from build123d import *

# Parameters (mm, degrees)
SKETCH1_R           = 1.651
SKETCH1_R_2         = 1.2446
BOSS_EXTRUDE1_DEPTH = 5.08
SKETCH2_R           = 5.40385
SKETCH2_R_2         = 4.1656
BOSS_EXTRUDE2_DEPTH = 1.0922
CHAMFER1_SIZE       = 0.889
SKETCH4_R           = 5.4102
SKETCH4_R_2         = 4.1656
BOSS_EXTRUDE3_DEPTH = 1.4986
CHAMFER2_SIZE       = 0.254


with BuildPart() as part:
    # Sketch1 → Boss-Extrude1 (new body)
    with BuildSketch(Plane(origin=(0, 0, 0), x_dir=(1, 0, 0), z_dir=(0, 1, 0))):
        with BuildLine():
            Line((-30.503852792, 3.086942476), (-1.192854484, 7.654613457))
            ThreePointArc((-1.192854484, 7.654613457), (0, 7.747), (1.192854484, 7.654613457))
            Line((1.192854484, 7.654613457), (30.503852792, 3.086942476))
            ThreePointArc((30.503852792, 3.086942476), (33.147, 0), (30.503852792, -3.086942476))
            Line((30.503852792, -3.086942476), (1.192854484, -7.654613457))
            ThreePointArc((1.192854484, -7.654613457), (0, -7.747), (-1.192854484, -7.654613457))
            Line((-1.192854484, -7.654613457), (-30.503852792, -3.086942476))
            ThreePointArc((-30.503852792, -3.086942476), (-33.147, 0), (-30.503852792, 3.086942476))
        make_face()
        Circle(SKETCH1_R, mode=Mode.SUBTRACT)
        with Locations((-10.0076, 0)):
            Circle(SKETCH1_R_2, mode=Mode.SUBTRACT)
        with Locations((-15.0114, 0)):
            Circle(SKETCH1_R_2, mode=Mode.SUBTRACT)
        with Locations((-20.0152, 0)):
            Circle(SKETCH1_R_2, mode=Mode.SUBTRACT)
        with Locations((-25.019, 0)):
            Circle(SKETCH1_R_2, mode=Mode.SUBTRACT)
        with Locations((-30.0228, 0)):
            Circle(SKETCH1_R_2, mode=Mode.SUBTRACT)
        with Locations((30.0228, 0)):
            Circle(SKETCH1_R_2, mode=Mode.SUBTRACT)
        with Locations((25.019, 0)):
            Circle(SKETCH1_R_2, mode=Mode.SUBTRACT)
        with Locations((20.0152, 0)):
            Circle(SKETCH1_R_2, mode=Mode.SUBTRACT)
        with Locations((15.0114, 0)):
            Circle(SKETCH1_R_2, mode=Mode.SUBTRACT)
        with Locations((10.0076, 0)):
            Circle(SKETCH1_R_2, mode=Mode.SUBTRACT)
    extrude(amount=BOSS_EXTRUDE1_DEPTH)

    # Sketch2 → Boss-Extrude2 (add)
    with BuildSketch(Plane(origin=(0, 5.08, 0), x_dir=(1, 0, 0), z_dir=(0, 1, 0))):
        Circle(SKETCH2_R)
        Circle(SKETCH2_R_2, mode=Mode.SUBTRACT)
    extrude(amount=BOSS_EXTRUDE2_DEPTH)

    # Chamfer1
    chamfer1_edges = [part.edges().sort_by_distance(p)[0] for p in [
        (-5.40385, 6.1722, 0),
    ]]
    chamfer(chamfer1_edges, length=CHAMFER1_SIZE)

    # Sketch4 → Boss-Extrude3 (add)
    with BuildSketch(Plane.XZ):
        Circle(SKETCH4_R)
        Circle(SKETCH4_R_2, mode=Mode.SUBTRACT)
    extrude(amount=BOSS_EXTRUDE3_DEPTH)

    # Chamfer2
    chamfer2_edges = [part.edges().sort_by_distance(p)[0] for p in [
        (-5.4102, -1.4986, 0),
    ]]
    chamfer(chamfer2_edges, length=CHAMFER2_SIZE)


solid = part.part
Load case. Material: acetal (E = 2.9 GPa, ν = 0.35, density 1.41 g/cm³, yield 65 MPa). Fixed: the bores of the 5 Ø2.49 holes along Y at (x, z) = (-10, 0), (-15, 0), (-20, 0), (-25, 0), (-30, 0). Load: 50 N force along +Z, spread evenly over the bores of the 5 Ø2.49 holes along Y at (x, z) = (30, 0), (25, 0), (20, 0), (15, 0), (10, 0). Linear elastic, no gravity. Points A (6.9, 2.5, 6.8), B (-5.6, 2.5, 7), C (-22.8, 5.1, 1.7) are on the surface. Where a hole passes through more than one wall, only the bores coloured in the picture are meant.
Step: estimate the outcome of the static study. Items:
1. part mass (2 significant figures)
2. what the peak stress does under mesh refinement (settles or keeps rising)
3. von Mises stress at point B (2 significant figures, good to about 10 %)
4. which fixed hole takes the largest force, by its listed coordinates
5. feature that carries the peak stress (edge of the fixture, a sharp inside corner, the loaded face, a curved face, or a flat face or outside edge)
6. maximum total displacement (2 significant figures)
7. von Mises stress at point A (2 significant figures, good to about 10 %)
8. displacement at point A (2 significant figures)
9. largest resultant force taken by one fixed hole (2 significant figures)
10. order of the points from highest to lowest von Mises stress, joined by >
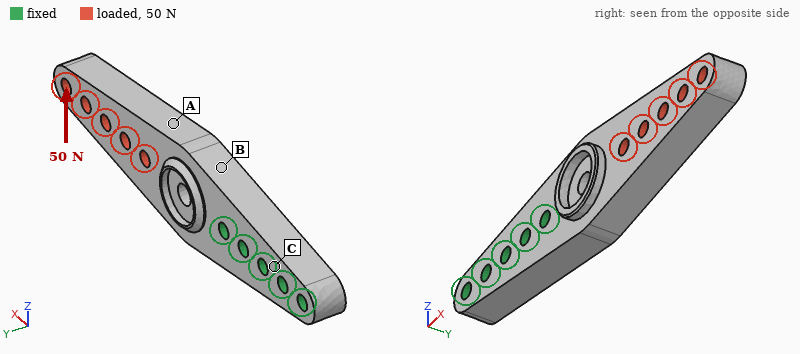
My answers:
4.7 g
keeps rising
8.1 MPa
(-10, 0)
edge of the fixture
0.43 mm
4.4 MPa
0.14 mm
180 N
B > A > C
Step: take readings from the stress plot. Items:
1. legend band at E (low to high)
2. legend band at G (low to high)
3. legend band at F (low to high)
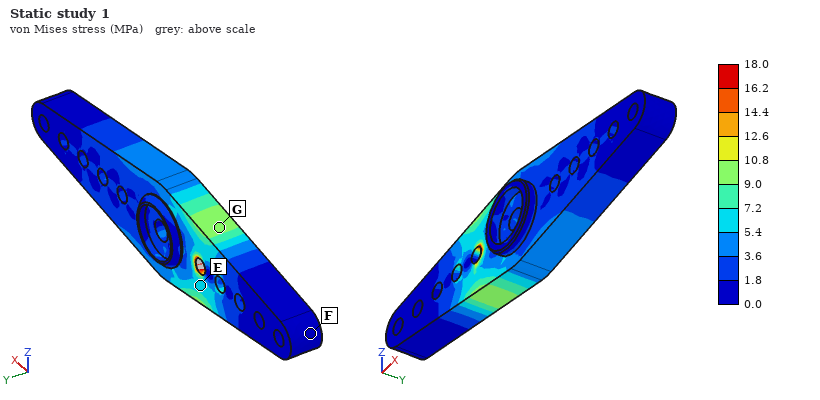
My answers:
5.4 to 7.2 MPa
9.0 to 10.8 MPa
0.0 to 1.8 MPa
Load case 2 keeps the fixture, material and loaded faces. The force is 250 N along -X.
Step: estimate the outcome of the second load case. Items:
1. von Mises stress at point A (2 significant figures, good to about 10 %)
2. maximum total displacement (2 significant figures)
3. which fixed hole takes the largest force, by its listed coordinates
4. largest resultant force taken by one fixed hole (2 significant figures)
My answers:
4.1 MPa
55 µm
(-10, 0)
180 N
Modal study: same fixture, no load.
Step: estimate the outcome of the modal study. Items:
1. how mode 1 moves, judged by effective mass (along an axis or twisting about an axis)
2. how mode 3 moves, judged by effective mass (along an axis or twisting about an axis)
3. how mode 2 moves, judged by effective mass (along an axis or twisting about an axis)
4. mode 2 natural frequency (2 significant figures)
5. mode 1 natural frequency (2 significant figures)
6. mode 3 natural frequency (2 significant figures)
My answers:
along Y
along Y
along Z
1700 Hz
860 Hz
3900 Hz
